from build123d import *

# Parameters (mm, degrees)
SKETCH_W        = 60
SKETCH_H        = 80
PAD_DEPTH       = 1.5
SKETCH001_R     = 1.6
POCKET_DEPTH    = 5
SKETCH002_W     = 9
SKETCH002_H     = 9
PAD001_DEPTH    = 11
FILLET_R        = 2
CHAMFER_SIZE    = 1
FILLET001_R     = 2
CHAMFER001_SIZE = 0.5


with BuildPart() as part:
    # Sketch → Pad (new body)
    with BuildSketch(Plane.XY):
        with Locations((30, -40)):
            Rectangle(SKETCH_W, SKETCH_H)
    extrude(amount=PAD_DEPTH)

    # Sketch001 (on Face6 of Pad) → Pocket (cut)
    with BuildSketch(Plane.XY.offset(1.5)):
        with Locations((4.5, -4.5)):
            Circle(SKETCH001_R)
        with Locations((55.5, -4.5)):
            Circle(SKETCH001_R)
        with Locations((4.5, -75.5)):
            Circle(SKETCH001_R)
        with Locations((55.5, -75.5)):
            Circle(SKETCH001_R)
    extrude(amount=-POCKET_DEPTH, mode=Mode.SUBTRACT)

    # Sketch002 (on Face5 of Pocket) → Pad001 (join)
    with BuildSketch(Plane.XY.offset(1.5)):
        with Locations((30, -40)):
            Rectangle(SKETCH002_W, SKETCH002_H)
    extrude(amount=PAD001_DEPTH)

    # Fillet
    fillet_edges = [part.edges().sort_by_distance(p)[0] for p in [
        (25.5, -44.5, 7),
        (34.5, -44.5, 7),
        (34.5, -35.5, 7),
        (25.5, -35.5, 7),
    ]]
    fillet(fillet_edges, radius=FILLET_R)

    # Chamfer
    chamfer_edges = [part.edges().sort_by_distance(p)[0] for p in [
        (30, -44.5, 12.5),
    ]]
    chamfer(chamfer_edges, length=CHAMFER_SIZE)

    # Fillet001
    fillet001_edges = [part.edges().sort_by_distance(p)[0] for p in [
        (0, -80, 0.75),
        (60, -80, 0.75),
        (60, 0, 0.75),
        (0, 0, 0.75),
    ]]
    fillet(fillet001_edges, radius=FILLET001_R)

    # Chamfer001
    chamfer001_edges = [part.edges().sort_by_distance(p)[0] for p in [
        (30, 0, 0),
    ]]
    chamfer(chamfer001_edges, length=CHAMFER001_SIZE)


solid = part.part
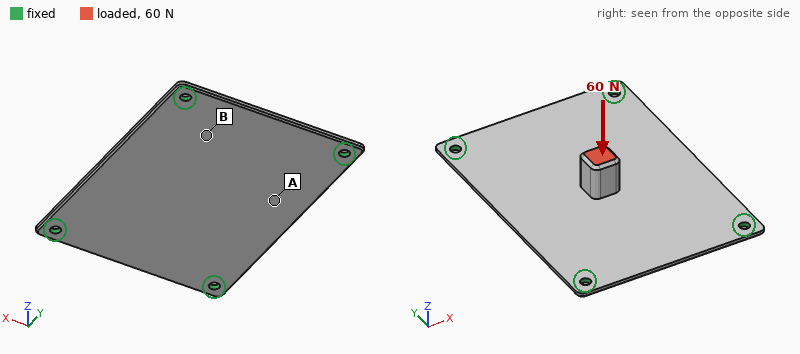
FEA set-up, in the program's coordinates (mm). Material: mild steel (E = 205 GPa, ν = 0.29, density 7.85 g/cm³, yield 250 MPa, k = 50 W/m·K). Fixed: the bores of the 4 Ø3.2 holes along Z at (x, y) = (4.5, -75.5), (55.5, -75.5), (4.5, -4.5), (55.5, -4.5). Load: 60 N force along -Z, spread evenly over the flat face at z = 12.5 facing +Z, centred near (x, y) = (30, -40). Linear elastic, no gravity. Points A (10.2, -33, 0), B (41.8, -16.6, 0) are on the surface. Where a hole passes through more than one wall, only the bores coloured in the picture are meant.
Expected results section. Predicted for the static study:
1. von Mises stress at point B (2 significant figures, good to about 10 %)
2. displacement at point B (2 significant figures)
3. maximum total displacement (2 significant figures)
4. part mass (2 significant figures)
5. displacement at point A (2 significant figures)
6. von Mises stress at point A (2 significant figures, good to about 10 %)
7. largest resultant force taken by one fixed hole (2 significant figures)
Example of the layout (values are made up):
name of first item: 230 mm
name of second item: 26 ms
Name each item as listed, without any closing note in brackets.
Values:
von Mises stress at point B: 6.3 MPa
displacement at point B: 20 µm
maximum total displacement: 49 µm
part mass: 62 g
displacement at point A: 35 µm
von Mises stress at point A: 14 MPa
largest resultant force taken by one fixed hole: 15 N
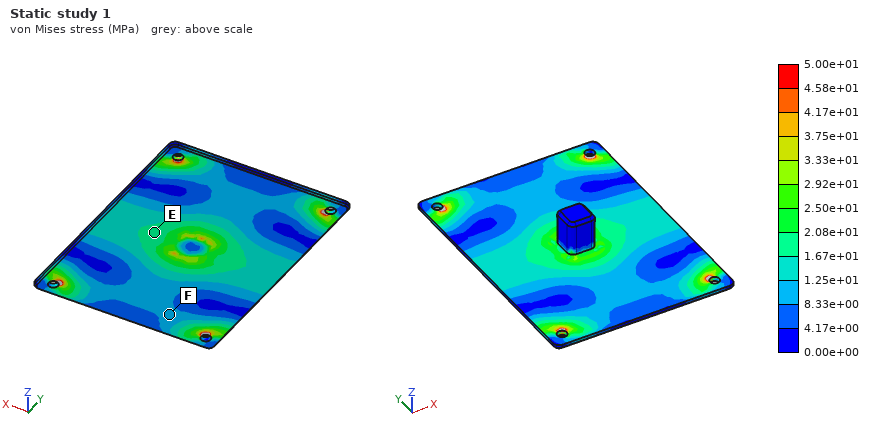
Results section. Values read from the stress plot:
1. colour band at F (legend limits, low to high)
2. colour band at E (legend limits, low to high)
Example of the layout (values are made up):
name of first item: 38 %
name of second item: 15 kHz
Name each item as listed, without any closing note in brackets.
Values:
colour band at F: 8.33e+00 to 1.25e+01 MPa
colour band at E: 1.67e+01 to 2.08e+01 MPa
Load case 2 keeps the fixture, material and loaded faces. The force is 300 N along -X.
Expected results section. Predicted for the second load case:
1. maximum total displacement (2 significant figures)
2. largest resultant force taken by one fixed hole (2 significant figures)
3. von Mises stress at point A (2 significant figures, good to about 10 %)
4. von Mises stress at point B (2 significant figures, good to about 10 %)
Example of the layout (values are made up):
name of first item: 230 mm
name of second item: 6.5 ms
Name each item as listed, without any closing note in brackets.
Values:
maximum total displacement: 0.10 mm
largest resultant force taken by one fixed hole: 100 N
von Mises stress at point A: 37 MPa
von Mises stress at point B: 33 MPa
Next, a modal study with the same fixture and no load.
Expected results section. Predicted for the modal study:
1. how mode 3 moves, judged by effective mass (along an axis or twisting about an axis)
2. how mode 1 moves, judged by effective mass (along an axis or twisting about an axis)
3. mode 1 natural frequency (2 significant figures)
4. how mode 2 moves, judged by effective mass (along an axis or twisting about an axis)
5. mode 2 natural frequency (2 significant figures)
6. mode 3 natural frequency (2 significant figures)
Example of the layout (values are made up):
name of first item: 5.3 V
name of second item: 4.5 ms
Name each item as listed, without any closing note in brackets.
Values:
how mode 3 moves, judged by effective mass: twisting about X
how mode 1 moves, judged by effective mass: along Z
mode 1 natural frequency: 1100 Hz
how mode 2 moves, judged by effective mass: twisting about Y
mode 2 natural frequency: 2000 Hz
mode 3 natural frequency: 2800 Hz
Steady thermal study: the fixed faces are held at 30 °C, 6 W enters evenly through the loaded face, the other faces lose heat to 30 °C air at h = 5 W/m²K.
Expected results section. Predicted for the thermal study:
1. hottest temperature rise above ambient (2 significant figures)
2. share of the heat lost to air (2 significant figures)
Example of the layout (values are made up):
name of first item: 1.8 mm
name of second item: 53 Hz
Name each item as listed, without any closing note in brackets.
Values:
hottest temperature rise above ambient: 58 K
share of the heat lost to air: 15 %
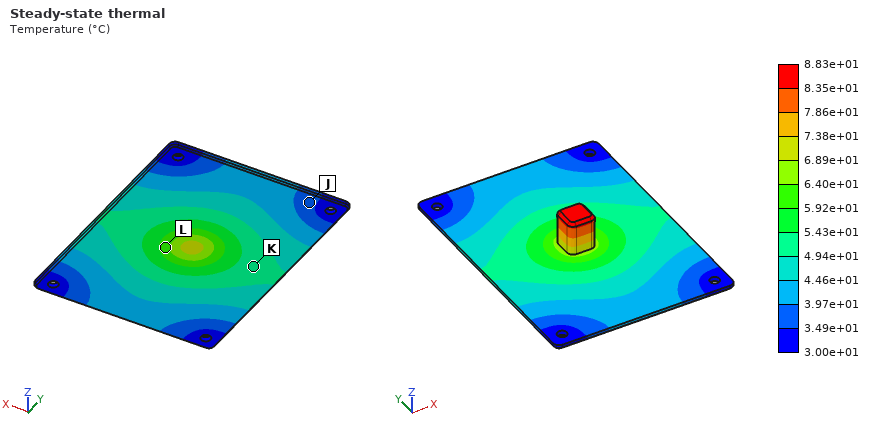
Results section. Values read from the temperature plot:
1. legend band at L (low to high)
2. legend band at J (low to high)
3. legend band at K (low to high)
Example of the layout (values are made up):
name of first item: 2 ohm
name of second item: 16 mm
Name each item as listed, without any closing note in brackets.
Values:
legend band at L: 5.92e+01 to 6.40e+01 °C
legend band at J: 3.49e+01 to 3.97e+01 °C
legend band at K: 4.94e+01 to 5.43e+01 °C
